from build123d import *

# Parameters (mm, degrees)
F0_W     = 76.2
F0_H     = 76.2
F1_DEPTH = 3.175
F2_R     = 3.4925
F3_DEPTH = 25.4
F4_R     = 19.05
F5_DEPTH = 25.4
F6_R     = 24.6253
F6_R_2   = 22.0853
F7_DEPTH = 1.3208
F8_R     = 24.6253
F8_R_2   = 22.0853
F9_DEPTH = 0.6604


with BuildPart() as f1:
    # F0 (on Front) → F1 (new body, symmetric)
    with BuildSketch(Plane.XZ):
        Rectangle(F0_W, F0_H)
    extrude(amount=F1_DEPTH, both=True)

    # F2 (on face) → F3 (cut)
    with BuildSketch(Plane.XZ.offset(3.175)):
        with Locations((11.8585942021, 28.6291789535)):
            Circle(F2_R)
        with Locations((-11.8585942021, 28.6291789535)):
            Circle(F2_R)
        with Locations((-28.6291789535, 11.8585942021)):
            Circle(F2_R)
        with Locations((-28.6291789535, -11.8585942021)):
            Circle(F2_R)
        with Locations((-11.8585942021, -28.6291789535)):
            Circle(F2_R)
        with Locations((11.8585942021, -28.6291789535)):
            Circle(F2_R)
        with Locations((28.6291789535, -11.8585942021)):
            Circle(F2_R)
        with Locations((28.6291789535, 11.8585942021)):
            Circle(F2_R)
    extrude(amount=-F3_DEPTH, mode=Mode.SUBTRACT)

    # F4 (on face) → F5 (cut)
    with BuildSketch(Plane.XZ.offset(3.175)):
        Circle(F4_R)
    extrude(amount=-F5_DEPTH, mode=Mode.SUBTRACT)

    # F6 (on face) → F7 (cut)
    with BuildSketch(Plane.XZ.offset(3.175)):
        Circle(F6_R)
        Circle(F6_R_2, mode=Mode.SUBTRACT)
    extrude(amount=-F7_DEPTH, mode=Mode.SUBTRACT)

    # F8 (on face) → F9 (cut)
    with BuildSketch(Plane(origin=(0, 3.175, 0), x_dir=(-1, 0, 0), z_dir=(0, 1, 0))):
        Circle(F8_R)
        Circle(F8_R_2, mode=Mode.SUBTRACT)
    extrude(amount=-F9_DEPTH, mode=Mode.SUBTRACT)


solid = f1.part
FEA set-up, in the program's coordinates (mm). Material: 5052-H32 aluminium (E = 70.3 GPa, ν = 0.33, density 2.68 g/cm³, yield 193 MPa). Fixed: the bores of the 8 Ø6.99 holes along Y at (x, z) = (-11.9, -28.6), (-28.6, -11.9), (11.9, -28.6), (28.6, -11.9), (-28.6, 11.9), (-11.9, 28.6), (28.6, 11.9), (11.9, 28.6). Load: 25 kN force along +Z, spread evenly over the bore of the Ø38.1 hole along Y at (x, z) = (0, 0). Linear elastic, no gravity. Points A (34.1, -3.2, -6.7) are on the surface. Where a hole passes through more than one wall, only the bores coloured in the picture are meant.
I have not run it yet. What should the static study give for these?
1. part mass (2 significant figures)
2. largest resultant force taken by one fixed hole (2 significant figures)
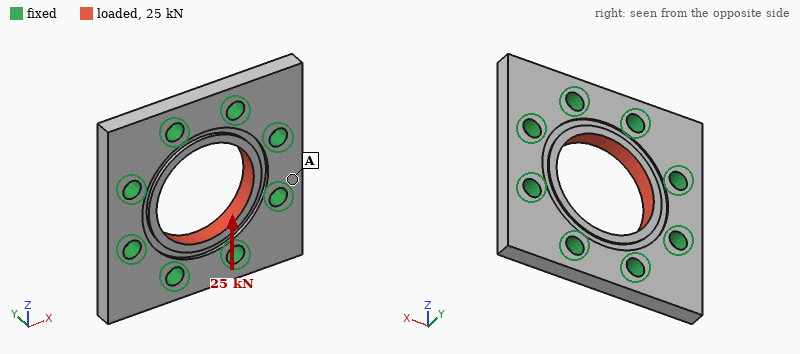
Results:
72 g
4.1 kN
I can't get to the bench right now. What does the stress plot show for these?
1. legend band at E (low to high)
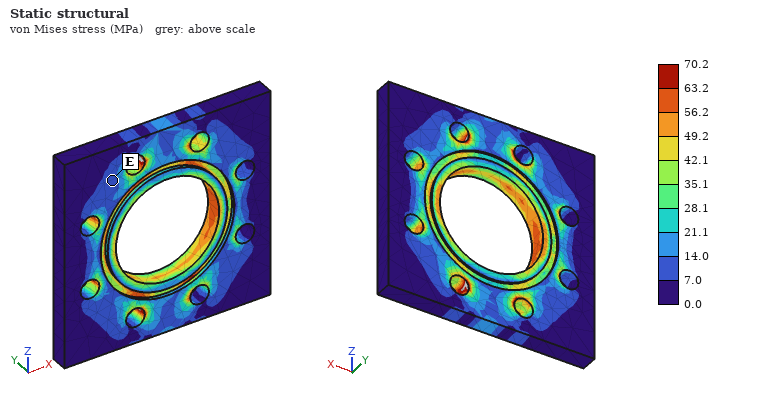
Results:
7.0 to 14.0 MPa
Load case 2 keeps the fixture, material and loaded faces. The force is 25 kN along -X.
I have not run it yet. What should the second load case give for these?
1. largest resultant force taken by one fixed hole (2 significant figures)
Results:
4.1 kN
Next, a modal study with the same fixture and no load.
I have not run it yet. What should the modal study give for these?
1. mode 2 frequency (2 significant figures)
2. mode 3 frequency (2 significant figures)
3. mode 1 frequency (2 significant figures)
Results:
15 kHz
15 kHz
15 kHz
